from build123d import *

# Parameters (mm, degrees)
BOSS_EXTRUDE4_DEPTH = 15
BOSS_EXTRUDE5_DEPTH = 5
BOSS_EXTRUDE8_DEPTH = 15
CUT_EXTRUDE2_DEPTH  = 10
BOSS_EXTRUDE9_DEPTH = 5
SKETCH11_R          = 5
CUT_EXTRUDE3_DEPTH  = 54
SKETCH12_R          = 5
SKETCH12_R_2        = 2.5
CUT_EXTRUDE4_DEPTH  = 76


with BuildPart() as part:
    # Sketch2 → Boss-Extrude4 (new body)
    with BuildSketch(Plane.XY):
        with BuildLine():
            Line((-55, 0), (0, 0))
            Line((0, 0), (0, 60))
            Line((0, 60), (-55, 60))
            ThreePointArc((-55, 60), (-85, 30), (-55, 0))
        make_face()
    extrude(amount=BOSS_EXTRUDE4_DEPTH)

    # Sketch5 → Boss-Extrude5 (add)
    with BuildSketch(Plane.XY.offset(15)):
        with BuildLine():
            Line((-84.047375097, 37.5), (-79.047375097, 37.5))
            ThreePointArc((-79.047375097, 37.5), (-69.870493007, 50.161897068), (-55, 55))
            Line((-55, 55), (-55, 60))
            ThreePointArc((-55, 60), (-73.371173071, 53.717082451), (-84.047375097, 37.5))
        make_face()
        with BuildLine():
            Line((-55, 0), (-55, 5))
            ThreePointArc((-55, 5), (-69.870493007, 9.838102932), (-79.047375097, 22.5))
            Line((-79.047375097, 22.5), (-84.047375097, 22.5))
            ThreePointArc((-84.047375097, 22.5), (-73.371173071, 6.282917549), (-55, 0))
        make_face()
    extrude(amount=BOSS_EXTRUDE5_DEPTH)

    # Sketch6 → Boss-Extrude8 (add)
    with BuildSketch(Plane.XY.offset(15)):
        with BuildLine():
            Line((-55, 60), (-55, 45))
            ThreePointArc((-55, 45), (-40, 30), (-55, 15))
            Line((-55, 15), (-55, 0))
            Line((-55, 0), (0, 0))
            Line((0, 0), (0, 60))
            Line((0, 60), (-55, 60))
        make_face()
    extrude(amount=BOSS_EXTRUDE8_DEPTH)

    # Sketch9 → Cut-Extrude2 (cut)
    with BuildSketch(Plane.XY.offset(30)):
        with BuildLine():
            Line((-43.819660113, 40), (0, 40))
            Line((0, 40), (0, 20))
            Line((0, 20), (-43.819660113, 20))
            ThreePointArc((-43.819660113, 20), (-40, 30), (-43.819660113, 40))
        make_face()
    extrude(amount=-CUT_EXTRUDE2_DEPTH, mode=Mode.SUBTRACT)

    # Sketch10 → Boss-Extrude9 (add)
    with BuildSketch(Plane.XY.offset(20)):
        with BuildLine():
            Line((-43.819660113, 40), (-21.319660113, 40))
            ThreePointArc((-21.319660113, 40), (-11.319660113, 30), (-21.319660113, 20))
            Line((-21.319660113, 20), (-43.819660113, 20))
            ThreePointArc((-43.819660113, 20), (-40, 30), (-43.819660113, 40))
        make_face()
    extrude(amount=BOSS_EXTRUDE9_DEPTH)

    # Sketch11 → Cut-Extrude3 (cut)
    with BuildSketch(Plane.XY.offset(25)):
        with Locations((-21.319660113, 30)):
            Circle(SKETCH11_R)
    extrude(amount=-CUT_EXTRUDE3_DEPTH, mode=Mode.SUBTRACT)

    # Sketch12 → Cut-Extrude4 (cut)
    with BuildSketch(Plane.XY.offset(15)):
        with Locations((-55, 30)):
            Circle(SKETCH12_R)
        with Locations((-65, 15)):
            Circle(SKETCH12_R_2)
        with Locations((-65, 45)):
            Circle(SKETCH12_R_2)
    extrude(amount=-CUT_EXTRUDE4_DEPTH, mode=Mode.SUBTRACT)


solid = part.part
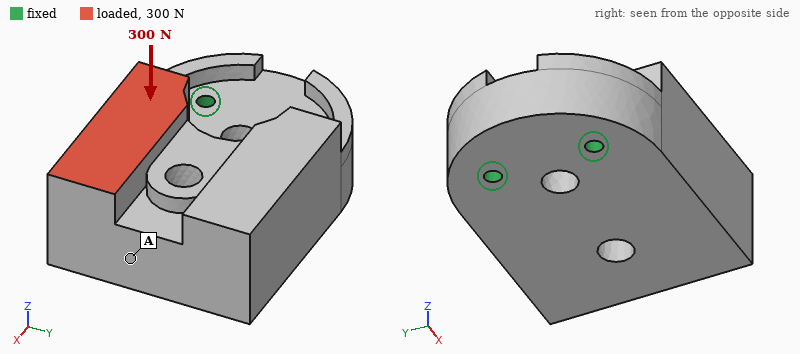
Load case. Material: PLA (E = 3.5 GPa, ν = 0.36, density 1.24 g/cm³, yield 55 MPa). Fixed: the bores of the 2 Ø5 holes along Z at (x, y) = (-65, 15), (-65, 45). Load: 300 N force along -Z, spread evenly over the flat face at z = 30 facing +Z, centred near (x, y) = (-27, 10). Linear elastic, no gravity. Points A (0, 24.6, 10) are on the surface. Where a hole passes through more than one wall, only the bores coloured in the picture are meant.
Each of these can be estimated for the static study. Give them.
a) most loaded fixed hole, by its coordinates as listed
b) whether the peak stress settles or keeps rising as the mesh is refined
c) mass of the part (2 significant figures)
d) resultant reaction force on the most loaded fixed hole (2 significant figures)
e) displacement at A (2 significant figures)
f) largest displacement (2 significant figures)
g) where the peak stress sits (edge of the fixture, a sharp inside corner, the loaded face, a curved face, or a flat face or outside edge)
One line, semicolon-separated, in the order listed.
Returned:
(-65, 15); keeps rising; 130 g; 290 N; 0.22 mm; 0.27 mm; edge of the fixture
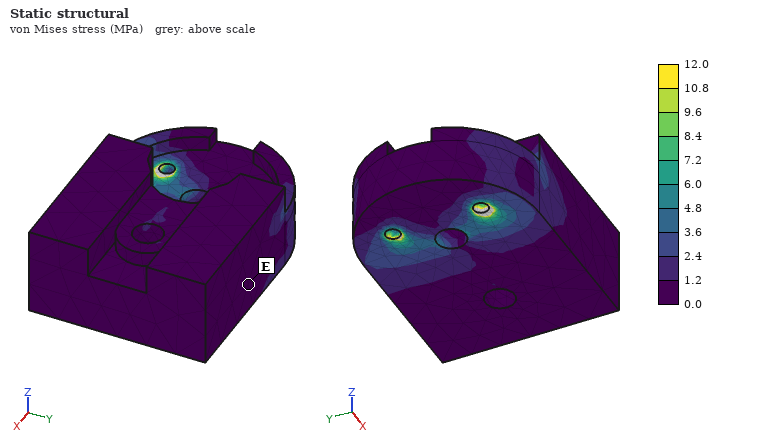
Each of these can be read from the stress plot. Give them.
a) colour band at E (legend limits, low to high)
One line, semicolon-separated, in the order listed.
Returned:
0.0 to 1.2 MPa
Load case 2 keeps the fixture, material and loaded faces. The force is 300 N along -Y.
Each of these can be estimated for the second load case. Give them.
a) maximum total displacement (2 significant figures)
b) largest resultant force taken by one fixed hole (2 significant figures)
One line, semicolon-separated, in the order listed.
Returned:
86 µm; 400 N
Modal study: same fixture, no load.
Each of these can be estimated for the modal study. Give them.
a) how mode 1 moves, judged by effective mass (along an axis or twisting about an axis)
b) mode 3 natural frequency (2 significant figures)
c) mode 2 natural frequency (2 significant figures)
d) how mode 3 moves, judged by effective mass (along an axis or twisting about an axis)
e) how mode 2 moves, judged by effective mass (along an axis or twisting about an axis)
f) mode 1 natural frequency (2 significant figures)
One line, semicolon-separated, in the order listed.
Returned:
along Z; 1800 Hz; 1500 Hz; twisting about X; along Y; 680 Hz
